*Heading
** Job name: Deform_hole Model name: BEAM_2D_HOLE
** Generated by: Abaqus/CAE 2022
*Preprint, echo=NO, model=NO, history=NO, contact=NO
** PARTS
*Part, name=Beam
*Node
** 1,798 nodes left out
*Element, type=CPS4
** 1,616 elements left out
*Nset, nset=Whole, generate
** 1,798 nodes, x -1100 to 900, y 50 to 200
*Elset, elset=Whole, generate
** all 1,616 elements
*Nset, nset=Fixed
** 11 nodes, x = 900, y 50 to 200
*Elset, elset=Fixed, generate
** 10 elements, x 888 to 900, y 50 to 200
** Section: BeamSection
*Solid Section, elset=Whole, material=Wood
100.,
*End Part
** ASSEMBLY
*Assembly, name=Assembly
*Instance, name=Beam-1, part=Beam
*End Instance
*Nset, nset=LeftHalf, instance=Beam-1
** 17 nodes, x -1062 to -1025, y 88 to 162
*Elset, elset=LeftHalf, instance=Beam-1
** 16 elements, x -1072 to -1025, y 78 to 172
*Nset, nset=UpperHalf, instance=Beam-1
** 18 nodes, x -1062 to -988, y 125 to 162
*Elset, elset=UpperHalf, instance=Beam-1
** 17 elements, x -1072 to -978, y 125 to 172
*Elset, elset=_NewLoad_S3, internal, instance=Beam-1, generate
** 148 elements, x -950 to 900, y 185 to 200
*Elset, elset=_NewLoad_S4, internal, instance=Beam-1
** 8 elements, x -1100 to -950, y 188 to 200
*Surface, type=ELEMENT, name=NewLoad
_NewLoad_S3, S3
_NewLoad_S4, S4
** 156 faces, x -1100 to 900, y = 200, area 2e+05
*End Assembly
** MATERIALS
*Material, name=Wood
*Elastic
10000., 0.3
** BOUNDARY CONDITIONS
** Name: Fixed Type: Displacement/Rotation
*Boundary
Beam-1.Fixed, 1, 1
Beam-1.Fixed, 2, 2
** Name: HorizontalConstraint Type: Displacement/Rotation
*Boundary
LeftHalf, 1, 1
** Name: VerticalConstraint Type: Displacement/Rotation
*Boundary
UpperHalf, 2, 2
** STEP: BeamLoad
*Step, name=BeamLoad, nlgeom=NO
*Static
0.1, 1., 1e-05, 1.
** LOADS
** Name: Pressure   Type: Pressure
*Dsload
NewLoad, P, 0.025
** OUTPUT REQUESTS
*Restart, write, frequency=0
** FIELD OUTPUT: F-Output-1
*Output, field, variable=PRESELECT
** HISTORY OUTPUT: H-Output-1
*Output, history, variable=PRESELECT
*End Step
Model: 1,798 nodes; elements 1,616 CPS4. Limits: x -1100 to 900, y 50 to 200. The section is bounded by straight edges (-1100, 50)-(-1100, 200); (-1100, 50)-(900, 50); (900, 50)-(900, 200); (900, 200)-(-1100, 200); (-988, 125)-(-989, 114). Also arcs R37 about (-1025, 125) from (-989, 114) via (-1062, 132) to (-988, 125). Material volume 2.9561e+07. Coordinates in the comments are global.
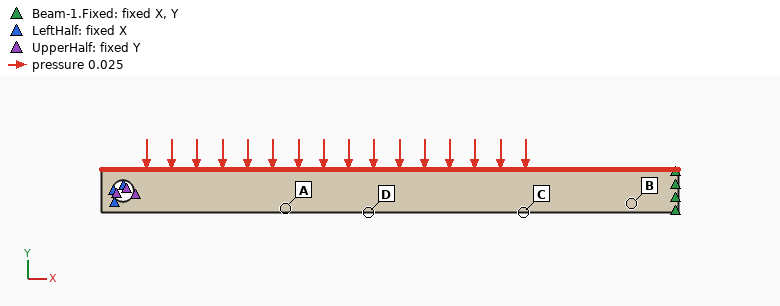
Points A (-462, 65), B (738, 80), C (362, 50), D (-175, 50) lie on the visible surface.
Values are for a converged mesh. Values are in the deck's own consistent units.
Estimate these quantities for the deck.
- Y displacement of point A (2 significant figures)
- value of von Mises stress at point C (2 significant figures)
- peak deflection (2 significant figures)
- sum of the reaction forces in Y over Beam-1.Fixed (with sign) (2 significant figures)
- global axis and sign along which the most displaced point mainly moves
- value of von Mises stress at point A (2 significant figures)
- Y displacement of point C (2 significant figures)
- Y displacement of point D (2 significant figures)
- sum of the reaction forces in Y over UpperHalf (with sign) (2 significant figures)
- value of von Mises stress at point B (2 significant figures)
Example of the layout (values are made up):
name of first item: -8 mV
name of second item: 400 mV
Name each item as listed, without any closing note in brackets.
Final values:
Y displacement of point A: -0.27
value of von Mises stress at point C: 0.41
peak deflection: 0.37
sum of the reaction forces in Y over Beam-1.Fixed (with sign): 2500
global axis and sign along which the most displaced point mainly moves: -Y
value of von Mises stress at point A: 0.49
Y displacement of point C: -0.23
Y displacement of point D: -0.36
sum of the reaction forces in Y over UpperHalf (with sign): 2500
value of von Mises stress at point B: 0.73
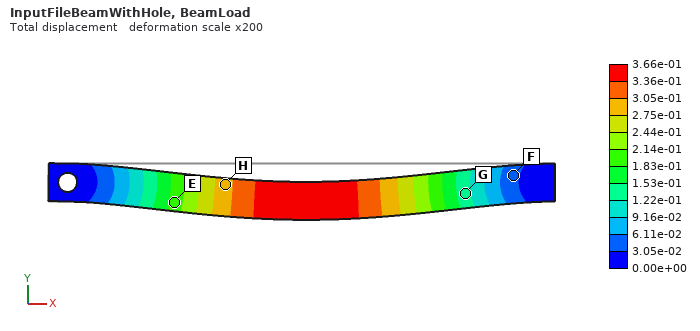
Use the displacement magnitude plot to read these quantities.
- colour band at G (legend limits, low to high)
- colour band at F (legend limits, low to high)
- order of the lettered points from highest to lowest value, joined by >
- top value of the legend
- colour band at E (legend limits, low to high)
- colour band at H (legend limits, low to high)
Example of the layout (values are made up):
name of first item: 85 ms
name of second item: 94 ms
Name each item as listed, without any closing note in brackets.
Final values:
colour band at G: 1.22e-01 to 1.53e-01
colour band at F: 3.05e-02 to 6.11e-02
order of the lettered points from highest to lowest value, joined by >: H > E > G > F
top value of the legend: 3.66e-01
colour band at E: 1.83e-01 to 2.14e-01
colour band at H: 2.75e-01 to 3.05e-01
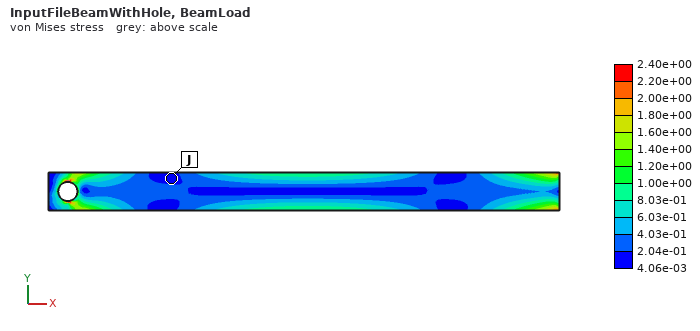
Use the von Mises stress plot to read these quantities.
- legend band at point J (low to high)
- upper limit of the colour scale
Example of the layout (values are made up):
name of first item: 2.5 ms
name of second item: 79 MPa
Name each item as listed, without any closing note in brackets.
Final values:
legend band at point J: 4.06e-03 to 2.04e-01
upper limit of the colour scale: 2.40e+00
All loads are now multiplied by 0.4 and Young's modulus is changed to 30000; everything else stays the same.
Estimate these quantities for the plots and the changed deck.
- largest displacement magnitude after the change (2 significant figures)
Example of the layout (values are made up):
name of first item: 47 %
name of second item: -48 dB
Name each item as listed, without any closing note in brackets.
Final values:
largest displacement magnitude after the change: 0.049
